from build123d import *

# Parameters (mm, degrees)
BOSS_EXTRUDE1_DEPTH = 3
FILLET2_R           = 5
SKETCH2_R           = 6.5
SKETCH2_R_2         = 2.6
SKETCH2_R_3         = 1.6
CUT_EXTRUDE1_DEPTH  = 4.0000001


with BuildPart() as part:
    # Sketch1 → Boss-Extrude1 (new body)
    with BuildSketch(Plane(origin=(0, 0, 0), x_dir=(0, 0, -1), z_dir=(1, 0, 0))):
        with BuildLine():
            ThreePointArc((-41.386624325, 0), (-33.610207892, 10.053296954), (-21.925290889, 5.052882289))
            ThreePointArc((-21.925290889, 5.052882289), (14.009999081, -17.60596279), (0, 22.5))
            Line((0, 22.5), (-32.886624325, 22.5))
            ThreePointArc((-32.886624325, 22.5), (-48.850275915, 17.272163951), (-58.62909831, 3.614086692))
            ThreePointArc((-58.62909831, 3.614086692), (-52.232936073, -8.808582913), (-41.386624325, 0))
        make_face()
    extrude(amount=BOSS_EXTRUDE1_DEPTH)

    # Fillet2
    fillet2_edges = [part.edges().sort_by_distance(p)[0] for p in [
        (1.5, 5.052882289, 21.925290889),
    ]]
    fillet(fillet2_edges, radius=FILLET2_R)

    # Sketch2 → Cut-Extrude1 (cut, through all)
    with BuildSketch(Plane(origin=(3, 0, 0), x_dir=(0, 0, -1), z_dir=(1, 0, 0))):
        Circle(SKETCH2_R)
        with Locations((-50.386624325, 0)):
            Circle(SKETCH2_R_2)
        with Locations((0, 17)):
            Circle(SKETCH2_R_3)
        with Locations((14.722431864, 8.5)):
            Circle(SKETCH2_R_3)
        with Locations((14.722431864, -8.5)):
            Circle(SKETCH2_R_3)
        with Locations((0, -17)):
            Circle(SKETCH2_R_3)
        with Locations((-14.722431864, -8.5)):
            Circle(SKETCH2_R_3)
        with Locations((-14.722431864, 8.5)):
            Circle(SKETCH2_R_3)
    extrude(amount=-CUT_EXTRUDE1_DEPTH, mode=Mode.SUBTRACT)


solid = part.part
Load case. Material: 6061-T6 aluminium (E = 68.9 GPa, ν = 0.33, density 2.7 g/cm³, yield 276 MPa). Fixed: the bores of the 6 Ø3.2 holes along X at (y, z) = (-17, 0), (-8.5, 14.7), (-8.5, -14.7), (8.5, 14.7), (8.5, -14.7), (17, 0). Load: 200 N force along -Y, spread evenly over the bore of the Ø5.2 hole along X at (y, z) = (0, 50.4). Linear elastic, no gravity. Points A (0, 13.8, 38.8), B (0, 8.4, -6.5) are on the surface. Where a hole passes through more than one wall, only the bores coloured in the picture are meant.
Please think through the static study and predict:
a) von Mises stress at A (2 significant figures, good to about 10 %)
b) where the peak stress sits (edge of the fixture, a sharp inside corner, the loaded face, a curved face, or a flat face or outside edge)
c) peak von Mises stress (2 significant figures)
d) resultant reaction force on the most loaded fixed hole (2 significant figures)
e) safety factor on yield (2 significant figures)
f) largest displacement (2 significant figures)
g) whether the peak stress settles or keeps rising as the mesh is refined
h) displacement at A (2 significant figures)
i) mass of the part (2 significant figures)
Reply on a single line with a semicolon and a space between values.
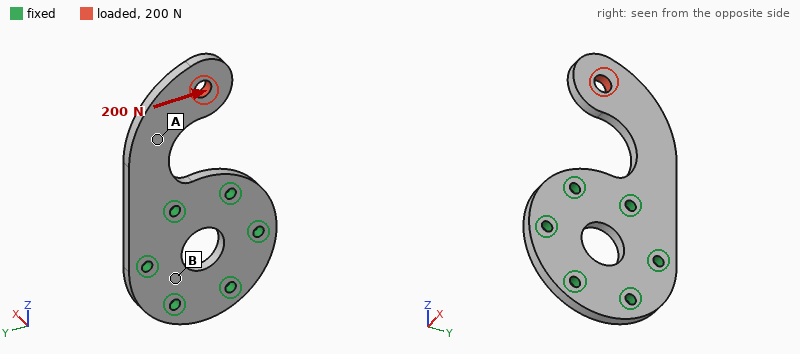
15 MPa; a curved face; 77 MPa; 320 N; 3.6; 0.11 mm; settles; 0.036 mm; 17 g
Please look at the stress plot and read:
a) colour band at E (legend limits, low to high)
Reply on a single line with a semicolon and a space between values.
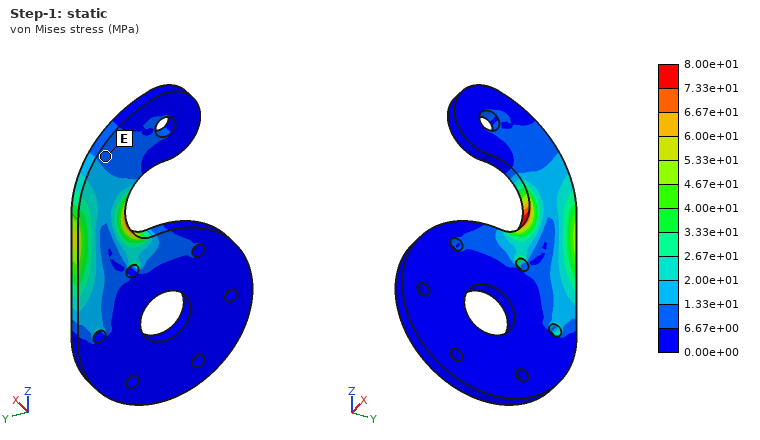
6.67e+00 to 1.33e+01 MPa
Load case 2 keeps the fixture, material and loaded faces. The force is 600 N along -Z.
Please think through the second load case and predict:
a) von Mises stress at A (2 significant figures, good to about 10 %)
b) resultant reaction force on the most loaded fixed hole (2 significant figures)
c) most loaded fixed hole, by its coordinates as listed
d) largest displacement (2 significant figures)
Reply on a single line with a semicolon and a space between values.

31 MPa; 650 N; (8.5, 14.7); 0.24 mm
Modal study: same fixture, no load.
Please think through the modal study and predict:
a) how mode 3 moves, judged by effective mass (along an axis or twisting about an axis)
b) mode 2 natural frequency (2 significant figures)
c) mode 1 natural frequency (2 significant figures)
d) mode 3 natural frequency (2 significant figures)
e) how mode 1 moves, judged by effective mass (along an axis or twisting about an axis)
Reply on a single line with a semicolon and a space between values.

along Y; 3200 Hz; 1000 Hz; 4200 Hz; along X
